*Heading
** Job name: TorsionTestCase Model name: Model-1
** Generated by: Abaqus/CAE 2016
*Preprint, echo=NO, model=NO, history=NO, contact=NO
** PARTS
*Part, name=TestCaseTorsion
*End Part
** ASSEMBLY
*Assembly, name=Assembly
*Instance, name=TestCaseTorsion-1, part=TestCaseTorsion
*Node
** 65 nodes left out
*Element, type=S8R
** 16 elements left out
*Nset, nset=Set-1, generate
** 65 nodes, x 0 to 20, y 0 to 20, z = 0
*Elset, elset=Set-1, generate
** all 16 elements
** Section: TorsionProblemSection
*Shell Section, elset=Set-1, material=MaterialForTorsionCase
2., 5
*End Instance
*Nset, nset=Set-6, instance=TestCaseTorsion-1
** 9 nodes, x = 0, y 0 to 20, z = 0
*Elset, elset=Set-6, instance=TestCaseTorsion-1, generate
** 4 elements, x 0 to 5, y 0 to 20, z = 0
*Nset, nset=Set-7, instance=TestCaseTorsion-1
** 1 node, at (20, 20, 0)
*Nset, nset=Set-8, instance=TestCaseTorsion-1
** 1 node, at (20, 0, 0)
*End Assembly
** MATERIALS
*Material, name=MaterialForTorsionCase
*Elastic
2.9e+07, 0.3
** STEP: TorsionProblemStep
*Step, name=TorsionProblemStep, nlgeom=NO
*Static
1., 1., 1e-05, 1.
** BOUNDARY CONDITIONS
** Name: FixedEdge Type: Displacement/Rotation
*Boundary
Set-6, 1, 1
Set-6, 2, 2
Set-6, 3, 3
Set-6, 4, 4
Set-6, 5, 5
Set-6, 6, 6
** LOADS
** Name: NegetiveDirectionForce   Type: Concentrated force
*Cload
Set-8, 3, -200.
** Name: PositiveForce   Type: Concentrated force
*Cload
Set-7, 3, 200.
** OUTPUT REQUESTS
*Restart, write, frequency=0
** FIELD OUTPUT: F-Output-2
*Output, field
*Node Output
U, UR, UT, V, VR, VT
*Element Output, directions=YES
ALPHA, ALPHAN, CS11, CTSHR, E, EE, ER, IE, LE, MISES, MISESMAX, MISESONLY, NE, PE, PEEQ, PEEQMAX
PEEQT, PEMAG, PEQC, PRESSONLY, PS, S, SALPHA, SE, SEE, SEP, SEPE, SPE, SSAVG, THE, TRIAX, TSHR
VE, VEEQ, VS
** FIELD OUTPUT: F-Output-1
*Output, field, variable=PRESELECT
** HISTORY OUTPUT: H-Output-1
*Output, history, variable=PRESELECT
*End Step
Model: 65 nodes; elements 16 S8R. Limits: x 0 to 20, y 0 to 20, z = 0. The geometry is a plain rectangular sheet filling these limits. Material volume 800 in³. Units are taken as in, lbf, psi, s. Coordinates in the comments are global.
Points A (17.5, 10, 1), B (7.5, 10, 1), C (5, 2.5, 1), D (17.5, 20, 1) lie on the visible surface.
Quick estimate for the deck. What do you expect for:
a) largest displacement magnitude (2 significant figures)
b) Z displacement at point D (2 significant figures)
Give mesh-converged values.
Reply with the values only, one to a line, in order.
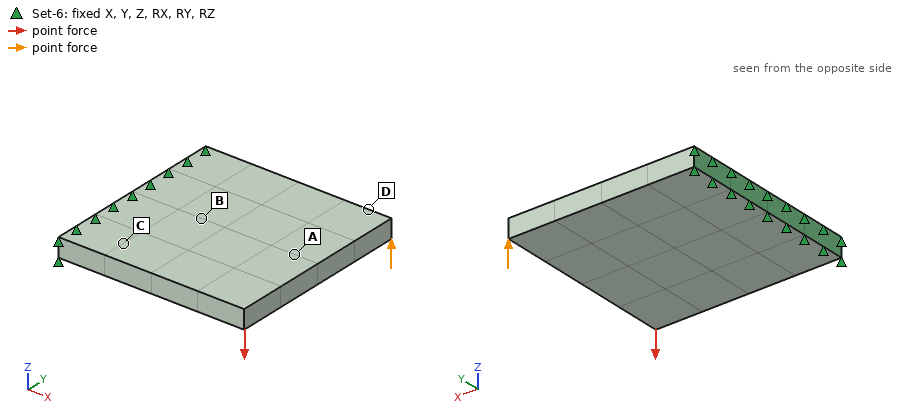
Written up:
0.0011 in
9.3e-04 in
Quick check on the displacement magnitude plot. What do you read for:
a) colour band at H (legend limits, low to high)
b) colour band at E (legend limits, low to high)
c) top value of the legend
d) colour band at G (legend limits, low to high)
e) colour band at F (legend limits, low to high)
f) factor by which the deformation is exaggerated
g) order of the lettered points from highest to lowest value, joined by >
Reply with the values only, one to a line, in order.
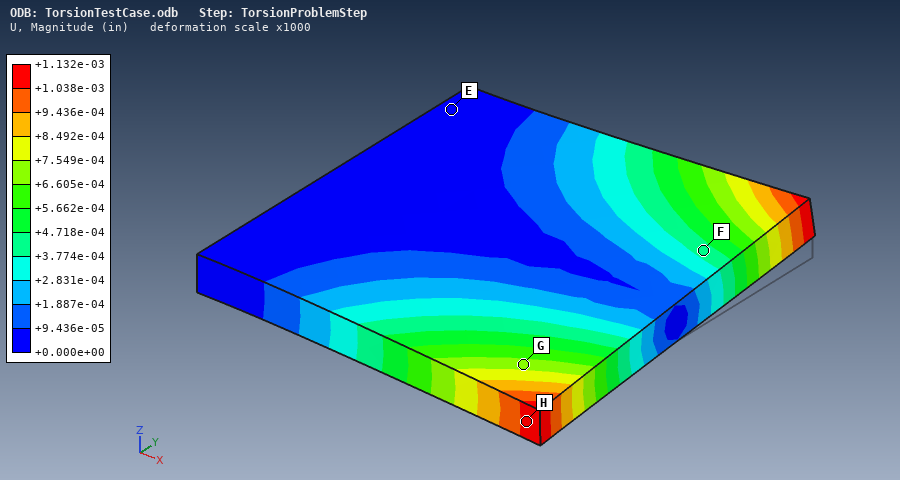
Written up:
+1.038e-03 to +1.132e-03 in
+0.000e+00 to +9.436e-05 in
+1.132e-03 in
+6.605e-04 to +7.549e-04 in
+3.774e-04 to +4.718e-04 in
1000
H > G > F > E
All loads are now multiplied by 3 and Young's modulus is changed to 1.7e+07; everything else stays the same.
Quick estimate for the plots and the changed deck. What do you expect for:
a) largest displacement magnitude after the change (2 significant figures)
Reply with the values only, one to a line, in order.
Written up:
0.0058 in
